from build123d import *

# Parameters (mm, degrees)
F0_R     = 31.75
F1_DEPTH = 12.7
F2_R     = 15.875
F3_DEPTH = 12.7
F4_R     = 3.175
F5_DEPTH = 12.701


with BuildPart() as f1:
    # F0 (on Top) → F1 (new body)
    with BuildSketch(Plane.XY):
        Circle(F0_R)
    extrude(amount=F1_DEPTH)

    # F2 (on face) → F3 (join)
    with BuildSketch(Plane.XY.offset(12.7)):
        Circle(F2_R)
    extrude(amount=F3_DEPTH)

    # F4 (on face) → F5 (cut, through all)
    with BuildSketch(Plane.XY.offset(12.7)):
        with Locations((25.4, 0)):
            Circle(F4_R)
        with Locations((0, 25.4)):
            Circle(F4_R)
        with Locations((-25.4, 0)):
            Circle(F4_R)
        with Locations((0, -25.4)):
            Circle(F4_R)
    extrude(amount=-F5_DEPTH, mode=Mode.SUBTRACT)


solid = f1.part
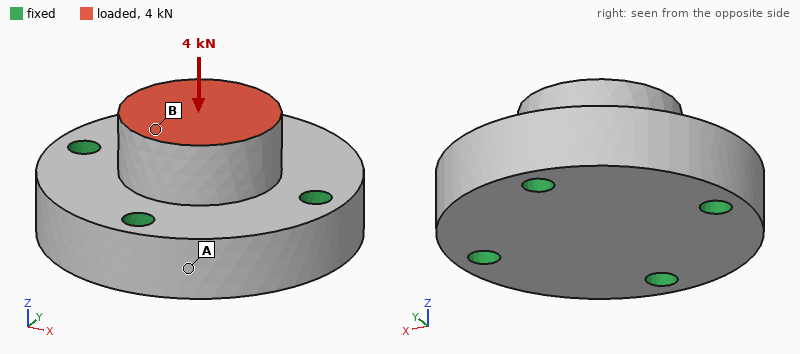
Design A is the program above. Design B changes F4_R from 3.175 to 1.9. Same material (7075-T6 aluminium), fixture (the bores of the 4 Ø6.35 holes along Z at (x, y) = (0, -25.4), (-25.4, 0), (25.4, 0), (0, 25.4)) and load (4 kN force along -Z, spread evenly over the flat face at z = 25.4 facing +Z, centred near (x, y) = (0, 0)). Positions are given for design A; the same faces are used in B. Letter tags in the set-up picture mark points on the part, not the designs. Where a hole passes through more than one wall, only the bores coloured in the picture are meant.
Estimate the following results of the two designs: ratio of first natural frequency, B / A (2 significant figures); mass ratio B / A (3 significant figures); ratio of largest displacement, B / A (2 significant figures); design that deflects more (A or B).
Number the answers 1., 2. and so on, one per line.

1. 0.87
2. 1.02
3. 1.2
4. B
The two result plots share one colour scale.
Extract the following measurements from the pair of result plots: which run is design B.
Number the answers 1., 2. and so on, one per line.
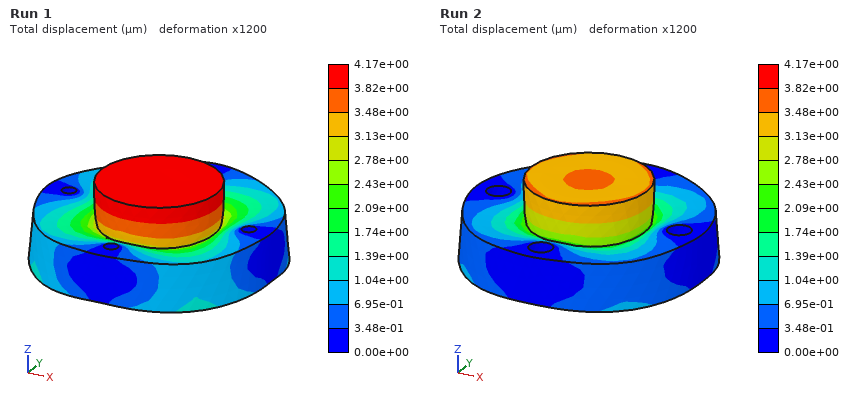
1. Run 1
